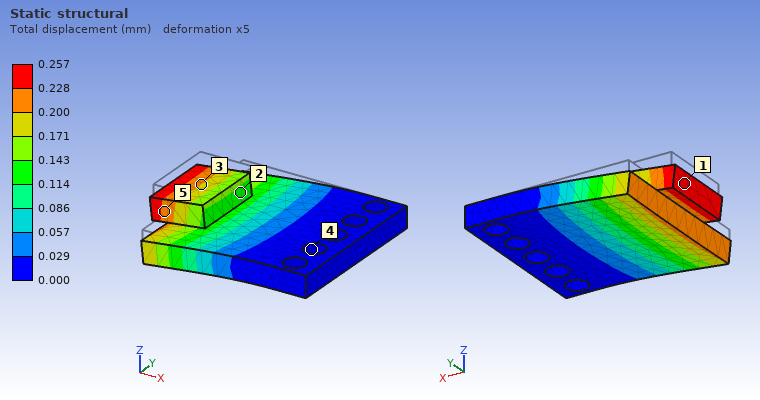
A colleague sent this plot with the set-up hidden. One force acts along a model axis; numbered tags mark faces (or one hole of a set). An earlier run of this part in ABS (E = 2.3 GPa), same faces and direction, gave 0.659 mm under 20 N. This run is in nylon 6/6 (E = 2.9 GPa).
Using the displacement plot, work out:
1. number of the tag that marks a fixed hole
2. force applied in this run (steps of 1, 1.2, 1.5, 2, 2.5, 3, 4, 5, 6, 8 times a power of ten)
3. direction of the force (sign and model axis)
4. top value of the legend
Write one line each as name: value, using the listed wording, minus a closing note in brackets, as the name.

number of the tag that marks a fixed hole: 4
force applied in this run: 10 N
direction of the force: -Z
top value of the legend: 0.257 mm
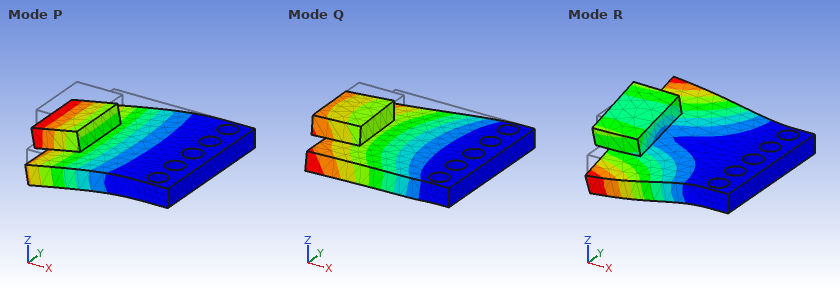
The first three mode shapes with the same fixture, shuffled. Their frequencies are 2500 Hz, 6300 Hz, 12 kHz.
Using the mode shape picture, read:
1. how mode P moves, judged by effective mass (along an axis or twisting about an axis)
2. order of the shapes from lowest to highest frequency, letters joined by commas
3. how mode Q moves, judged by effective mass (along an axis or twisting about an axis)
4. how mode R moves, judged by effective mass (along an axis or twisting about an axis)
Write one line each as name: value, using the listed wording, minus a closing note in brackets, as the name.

how mode P moves, judged by effective mass: along Z
order of the shapes from lowest to highest frequency, letters joined by commas: P, R, Q
how mode Q moves, judged by effective mass: along Y
how mode R moves, judged by effective mass: twisting about X
